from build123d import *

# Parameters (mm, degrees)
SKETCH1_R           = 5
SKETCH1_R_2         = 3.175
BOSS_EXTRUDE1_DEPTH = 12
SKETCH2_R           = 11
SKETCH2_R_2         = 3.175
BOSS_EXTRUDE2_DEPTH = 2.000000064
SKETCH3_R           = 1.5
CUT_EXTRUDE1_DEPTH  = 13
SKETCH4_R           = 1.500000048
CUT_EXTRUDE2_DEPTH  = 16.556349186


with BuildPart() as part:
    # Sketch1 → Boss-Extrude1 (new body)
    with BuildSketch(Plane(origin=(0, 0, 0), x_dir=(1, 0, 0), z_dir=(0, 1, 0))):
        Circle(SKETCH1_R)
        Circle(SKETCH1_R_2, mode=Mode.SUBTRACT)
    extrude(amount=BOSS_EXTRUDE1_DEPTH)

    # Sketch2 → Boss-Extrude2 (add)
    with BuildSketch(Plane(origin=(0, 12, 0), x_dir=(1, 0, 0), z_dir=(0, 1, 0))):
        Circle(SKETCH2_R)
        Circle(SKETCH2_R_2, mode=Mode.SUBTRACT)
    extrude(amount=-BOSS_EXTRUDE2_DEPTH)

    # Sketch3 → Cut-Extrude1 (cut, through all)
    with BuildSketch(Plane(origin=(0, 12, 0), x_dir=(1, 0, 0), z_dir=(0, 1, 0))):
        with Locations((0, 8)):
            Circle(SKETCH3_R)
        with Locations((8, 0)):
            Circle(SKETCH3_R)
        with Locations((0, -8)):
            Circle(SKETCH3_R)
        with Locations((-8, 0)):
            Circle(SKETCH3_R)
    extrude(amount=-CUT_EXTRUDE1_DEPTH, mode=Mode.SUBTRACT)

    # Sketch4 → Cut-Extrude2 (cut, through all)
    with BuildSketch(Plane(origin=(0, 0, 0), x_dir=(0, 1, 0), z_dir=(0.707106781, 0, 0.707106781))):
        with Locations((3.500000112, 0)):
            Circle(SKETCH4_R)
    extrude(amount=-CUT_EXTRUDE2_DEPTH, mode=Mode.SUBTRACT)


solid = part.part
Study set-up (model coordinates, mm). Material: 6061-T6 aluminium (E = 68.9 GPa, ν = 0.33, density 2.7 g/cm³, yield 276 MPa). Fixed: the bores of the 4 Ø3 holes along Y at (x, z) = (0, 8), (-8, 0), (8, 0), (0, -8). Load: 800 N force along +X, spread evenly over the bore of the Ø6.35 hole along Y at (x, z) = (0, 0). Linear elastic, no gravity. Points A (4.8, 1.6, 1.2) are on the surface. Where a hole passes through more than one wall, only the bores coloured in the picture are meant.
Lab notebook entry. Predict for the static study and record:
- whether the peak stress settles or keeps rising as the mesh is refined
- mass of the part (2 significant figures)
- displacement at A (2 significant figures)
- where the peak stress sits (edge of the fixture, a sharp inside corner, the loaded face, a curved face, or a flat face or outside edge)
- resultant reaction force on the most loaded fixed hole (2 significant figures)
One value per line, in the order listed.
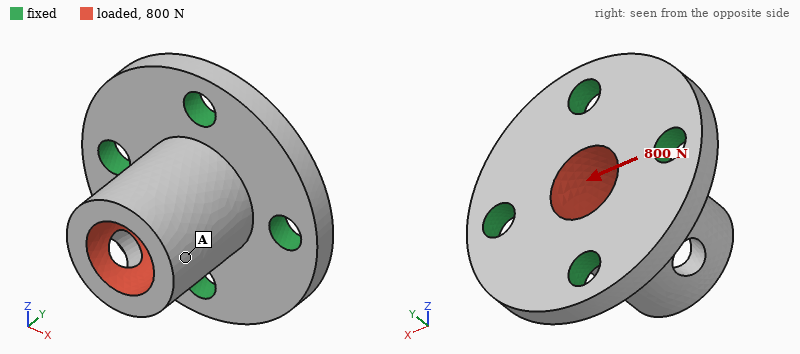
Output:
keeps rising
3.0 g
17 µm
edge of the fixture
400 N
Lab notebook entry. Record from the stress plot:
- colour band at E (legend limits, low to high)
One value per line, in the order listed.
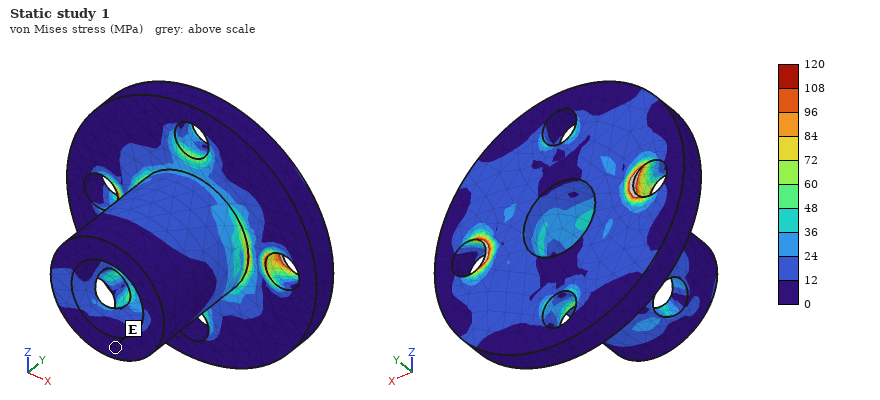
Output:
0 to 12 MPa
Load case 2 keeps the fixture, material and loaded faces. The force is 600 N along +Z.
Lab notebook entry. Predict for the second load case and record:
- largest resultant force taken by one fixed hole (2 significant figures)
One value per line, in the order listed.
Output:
300 N
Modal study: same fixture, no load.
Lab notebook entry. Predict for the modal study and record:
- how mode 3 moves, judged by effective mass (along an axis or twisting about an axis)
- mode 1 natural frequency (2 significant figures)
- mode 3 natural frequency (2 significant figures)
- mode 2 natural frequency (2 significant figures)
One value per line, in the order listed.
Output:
along Y
31 kHz
55 kHz
31 kHz
